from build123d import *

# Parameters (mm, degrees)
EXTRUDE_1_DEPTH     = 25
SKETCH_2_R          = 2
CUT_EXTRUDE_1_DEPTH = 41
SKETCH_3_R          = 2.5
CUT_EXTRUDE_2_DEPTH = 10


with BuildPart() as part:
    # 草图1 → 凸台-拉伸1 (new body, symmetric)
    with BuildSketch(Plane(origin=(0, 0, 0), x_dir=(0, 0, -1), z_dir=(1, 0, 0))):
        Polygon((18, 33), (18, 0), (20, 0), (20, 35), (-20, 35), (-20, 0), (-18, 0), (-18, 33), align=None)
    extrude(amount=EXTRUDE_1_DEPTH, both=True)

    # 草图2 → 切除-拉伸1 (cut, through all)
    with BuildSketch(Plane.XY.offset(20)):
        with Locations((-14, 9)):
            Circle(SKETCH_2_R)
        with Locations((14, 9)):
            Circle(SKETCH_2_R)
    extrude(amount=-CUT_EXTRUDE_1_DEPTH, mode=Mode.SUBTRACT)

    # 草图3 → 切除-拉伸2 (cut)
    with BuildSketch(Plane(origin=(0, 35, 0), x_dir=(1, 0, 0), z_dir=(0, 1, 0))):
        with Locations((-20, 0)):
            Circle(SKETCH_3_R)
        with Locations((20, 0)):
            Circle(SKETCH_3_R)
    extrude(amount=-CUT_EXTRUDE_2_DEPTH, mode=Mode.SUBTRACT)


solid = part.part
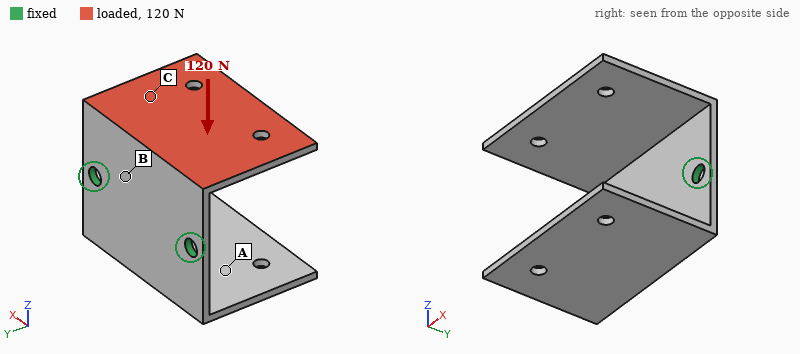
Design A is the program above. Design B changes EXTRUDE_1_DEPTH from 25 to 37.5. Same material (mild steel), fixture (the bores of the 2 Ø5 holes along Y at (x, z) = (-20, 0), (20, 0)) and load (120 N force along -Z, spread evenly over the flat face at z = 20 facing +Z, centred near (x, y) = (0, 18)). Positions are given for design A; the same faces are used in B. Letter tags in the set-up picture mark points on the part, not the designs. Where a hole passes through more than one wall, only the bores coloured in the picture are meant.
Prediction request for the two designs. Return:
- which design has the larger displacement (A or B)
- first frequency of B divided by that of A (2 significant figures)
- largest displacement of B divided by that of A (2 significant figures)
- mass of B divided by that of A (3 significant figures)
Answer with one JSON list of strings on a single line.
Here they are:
["A", "0.97", "0.68", "1.51"]
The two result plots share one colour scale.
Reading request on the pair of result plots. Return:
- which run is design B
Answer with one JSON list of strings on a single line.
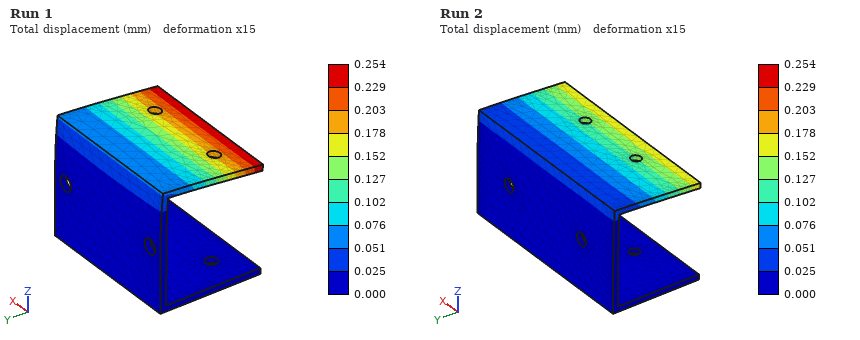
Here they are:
["Run 2"]
